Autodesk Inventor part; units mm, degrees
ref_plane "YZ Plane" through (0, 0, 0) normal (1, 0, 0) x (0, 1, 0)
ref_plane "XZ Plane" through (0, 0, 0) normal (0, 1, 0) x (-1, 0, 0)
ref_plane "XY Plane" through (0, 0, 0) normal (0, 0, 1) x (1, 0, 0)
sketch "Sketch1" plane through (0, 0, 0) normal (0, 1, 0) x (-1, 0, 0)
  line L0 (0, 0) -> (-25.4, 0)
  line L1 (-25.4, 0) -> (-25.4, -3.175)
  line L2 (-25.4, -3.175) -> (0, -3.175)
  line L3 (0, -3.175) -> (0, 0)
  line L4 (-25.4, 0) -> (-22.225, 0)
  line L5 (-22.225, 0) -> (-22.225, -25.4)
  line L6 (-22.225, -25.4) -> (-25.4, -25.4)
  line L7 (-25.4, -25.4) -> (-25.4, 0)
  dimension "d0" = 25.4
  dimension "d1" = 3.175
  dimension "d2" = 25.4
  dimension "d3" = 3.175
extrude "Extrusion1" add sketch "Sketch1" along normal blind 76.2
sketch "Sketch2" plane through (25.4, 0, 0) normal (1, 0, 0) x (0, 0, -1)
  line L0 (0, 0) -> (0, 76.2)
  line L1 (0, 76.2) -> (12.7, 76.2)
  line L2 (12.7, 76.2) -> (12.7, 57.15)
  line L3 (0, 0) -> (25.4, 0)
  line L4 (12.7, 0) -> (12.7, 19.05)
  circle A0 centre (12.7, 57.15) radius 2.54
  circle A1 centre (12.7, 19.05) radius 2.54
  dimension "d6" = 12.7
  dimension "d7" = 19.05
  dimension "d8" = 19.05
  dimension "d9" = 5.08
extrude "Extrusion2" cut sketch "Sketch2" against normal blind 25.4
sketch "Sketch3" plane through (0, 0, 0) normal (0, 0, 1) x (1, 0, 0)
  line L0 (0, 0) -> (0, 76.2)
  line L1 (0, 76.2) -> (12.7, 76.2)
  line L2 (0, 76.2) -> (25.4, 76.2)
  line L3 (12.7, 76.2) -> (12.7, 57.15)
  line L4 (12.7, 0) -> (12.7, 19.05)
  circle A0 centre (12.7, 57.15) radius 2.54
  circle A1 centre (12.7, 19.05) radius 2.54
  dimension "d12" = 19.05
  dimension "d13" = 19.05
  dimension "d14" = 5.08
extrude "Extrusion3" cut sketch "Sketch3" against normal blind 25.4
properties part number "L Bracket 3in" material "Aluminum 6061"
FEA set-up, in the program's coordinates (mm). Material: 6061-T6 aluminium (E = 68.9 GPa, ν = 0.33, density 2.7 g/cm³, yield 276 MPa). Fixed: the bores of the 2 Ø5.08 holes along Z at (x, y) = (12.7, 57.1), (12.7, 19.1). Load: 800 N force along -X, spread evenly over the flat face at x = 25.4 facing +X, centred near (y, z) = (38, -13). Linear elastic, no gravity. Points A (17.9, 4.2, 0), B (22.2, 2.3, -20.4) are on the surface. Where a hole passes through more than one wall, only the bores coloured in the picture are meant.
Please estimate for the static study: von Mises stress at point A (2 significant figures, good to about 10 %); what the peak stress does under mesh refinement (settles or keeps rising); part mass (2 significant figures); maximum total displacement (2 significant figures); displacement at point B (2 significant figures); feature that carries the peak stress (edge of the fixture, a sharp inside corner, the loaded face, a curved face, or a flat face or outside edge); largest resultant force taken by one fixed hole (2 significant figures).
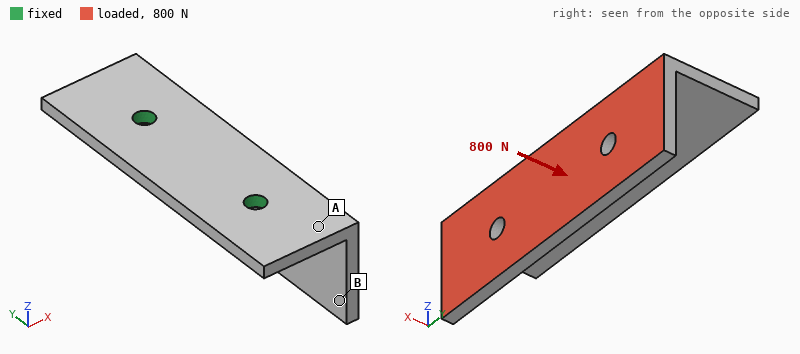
47 MPa
keeps rising
30 g
0.26 mm
0.19 mm
edge of the fixture
400 N
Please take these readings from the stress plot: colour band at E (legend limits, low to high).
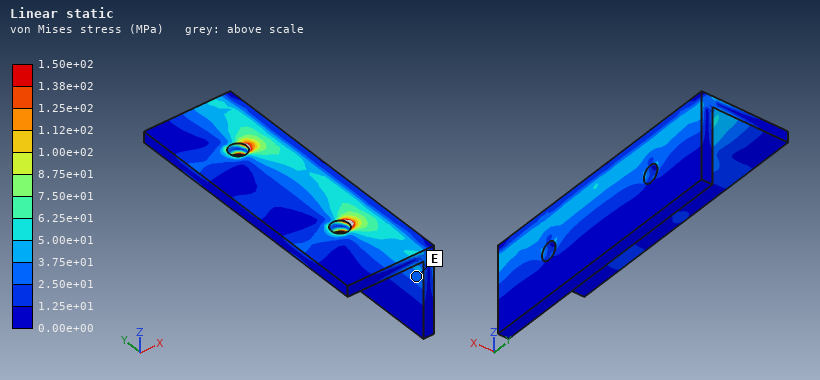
2.50e+01 to 3.75e+01 MPa
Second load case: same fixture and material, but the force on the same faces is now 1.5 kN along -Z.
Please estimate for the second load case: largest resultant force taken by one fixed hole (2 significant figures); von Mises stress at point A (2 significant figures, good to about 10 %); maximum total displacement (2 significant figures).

750 N
46 MPa
0.27 mm
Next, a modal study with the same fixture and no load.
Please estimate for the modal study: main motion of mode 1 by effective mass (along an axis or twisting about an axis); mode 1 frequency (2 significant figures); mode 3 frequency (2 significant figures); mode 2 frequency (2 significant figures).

along X
2600 Hz
6600 Hz
3600 Hz
